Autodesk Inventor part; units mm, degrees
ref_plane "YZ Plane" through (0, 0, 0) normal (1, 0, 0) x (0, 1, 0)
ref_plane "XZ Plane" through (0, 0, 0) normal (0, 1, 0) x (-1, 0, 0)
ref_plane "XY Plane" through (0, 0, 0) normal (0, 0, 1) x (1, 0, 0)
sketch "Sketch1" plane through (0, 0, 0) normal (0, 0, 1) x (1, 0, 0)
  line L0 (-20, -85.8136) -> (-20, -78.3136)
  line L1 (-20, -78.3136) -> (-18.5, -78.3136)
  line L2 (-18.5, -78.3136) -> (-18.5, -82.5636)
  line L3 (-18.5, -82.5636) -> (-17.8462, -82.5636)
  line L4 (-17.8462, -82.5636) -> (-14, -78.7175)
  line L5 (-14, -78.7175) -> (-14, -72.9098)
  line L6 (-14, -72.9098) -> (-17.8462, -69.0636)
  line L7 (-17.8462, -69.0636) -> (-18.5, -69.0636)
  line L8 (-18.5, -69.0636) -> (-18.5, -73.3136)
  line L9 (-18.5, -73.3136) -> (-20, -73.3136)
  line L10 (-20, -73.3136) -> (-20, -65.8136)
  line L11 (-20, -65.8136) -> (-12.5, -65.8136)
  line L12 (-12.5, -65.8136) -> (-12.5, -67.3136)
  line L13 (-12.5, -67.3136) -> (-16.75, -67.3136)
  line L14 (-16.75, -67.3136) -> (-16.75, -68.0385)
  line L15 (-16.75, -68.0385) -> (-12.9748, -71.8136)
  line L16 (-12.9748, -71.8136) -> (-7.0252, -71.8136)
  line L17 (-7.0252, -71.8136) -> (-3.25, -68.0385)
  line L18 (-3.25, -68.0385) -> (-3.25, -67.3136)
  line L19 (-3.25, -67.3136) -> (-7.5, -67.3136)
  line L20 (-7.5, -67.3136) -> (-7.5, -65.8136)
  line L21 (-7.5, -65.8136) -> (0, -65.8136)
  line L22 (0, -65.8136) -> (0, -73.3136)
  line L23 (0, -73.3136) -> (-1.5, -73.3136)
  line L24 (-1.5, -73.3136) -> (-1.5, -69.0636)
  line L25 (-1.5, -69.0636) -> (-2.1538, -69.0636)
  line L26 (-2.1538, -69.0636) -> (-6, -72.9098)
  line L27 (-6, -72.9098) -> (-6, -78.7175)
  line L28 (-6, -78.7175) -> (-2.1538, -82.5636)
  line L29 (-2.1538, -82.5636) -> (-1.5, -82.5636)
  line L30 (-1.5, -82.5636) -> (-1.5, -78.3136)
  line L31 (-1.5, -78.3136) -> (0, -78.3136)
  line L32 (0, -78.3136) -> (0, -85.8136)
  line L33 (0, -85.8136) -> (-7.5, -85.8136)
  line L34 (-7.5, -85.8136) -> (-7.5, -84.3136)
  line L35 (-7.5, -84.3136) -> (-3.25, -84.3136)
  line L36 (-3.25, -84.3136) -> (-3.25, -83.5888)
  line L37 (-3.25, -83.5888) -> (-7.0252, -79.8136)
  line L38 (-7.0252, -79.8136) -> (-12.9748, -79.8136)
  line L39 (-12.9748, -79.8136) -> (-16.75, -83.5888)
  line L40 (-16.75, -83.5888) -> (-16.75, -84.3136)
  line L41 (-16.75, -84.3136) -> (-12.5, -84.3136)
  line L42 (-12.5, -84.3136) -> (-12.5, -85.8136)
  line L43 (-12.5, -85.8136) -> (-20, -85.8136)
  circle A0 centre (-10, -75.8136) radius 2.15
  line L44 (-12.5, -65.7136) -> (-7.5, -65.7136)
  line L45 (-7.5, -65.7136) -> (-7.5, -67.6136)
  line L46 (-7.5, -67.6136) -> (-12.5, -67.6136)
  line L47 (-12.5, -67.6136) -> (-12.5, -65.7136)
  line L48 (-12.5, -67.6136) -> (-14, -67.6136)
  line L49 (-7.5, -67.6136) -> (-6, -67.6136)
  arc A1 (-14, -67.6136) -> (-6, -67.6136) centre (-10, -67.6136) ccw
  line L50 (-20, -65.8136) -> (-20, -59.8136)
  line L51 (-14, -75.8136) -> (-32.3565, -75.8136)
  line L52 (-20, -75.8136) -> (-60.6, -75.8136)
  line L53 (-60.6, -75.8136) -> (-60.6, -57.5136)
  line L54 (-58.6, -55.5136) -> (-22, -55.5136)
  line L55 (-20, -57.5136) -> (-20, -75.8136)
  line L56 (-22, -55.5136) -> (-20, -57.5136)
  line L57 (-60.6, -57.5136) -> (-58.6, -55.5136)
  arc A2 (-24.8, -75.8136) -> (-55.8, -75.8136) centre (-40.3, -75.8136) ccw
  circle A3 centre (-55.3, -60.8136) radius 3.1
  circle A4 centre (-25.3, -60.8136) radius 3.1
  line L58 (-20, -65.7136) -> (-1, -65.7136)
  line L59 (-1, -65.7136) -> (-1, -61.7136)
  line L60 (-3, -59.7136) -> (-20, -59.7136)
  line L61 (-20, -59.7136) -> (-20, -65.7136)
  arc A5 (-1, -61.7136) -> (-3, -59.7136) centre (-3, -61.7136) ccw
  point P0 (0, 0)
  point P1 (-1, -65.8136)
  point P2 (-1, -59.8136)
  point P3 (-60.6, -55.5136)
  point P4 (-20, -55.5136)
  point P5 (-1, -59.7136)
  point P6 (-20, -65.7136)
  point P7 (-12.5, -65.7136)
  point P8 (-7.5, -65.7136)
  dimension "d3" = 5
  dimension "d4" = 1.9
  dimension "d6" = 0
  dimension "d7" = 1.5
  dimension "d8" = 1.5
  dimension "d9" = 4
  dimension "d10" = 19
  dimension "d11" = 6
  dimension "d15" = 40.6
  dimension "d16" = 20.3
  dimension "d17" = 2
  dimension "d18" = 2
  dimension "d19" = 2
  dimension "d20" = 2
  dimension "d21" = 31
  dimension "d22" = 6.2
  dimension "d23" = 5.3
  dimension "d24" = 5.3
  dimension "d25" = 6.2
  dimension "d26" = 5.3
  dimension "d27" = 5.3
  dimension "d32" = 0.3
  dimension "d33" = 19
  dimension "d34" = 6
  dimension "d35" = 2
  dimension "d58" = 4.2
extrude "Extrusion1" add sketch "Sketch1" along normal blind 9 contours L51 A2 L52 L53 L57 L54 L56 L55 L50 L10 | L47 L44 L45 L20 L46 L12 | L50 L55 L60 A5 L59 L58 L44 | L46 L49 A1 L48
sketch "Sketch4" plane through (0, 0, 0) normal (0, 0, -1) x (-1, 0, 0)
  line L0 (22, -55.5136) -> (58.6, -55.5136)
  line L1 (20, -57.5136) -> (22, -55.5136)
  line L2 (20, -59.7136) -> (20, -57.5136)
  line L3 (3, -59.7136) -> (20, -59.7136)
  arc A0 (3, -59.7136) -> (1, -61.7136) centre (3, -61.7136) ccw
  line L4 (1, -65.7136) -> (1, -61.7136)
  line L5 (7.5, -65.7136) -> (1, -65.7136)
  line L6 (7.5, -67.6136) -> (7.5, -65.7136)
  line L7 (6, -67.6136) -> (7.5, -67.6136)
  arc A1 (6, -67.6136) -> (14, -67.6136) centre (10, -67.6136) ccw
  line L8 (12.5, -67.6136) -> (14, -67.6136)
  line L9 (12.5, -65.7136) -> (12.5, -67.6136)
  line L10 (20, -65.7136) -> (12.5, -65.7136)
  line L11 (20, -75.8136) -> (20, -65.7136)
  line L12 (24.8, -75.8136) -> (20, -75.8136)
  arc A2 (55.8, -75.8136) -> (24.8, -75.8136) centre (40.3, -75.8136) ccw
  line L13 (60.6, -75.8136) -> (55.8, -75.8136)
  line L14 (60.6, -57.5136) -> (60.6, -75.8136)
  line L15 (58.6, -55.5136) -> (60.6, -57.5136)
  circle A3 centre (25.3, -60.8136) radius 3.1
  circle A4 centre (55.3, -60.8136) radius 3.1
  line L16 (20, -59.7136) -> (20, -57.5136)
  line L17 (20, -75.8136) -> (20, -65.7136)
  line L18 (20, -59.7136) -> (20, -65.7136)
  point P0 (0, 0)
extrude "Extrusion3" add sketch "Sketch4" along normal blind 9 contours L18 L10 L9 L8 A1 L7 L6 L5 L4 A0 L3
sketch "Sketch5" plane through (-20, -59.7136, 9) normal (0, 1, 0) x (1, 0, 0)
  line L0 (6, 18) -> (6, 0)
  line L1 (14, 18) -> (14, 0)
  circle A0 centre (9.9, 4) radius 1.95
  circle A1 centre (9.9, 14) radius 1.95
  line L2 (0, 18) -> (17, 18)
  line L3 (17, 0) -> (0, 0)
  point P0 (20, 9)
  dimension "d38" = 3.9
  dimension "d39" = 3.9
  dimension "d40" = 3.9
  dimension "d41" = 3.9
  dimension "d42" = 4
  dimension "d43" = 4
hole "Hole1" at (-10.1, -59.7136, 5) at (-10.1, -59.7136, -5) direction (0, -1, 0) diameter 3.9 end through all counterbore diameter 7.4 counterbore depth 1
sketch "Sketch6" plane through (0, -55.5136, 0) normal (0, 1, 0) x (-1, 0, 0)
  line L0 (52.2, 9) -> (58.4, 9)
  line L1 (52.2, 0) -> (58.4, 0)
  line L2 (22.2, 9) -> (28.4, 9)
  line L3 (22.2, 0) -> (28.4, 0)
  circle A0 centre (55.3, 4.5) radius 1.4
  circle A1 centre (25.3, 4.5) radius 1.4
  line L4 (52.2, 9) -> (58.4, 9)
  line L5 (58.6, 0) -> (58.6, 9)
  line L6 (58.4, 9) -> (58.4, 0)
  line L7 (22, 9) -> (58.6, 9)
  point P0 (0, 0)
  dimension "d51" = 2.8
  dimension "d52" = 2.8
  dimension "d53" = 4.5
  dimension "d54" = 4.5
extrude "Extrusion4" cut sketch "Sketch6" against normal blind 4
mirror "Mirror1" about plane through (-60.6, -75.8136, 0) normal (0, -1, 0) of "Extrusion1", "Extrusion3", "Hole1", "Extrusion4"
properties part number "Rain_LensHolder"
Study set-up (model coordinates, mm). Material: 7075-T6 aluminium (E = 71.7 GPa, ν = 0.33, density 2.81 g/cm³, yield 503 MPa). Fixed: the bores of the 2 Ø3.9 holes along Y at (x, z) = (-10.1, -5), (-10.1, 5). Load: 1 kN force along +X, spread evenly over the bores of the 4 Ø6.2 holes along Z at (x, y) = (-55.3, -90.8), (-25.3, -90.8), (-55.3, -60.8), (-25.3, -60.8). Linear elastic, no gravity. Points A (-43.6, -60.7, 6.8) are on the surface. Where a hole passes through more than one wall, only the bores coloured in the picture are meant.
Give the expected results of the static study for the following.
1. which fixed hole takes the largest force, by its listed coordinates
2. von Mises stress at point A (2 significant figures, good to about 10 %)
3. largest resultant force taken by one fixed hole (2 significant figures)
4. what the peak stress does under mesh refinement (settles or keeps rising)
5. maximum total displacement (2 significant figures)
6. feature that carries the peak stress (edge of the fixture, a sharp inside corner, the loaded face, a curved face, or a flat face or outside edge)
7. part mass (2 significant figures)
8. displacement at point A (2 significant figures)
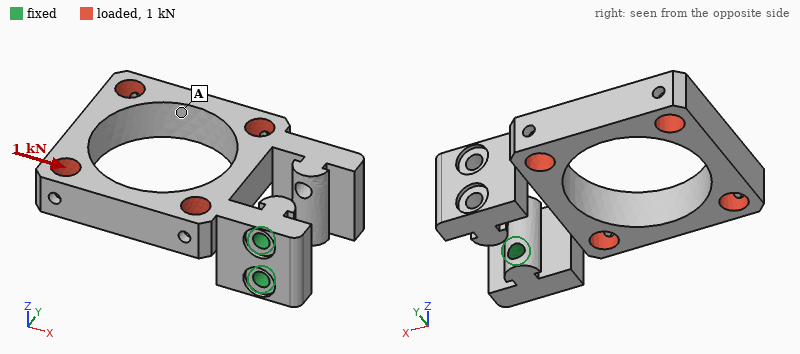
(-10.1, 5)
34 MPa
910 N
keeps rising
0.85 mm
a sharp inside corner
32 g
0.65 mm
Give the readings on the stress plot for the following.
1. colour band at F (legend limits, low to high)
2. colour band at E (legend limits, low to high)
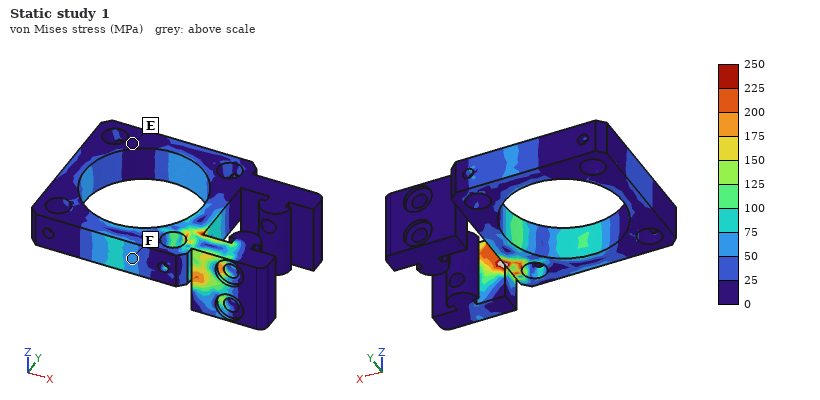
50 to 75 MPa
0 to 25 MPa
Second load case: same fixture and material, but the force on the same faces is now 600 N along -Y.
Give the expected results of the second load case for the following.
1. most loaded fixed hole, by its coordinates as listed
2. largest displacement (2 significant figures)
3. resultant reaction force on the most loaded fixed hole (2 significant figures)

(-10.1, 5)
0.83 mm
460 N
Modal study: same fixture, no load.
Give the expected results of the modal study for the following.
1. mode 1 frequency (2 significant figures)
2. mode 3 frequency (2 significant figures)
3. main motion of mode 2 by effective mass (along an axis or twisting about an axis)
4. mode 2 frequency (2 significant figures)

920 Hz
1700 Hz
along Z
1400 Hz
